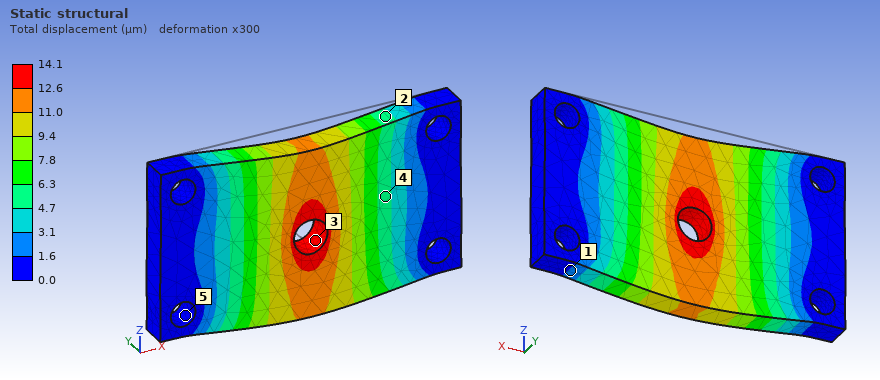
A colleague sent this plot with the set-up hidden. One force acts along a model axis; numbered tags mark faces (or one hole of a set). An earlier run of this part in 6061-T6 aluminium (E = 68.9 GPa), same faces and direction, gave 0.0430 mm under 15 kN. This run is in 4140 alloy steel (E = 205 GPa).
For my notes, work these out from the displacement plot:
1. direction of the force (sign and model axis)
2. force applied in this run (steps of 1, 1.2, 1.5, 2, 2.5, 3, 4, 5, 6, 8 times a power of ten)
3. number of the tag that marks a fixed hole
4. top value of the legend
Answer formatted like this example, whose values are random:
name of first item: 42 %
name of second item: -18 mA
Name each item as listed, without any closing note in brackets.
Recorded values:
direction of the force: -Z
force applied in this run: 15 kN
number of the tag that marks a fixed hole: 5
top value of the legend: 14.1 µm
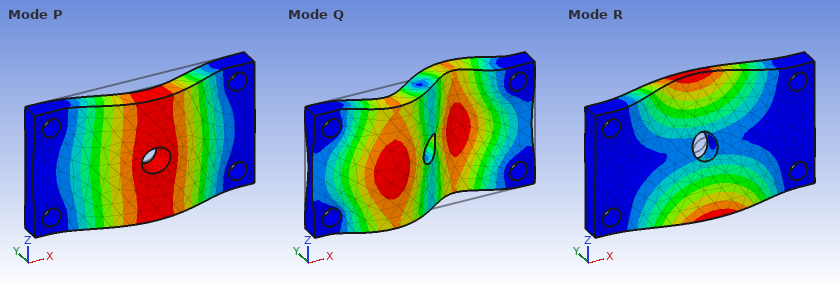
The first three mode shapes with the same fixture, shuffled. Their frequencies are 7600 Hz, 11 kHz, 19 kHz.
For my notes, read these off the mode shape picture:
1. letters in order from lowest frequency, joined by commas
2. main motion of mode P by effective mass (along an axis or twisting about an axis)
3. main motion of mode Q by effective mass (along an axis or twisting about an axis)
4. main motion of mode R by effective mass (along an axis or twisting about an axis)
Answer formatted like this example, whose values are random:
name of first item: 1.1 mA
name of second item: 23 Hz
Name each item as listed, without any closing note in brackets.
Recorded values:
letters in order from lowest frequency, joined by commas: P, R, Q
main motion of mode P by effective mass: along Y
main motion of mode Q by effective mass: twisting about Z
main motion of mode R by effective mass: twisting about X
